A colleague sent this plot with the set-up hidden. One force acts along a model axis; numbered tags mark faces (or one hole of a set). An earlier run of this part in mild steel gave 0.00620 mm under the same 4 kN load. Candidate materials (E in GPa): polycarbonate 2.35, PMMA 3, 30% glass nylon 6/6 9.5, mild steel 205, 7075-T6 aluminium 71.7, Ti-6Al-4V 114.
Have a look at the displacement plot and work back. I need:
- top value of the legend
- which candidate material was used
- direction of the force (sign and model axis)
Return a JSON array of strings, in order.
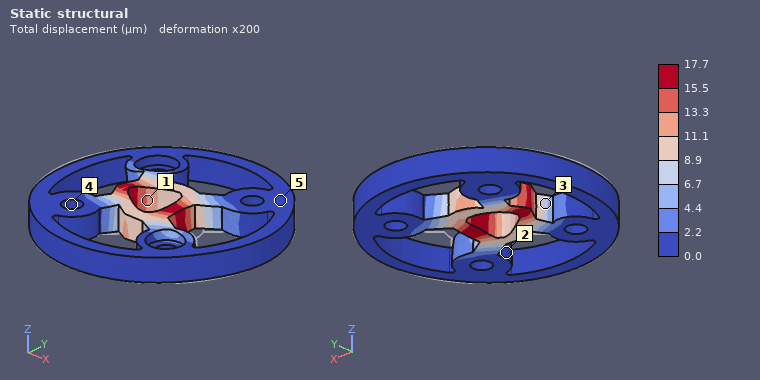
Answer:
["17.7 µm", "7075-T6 aluminium", "-X"]
